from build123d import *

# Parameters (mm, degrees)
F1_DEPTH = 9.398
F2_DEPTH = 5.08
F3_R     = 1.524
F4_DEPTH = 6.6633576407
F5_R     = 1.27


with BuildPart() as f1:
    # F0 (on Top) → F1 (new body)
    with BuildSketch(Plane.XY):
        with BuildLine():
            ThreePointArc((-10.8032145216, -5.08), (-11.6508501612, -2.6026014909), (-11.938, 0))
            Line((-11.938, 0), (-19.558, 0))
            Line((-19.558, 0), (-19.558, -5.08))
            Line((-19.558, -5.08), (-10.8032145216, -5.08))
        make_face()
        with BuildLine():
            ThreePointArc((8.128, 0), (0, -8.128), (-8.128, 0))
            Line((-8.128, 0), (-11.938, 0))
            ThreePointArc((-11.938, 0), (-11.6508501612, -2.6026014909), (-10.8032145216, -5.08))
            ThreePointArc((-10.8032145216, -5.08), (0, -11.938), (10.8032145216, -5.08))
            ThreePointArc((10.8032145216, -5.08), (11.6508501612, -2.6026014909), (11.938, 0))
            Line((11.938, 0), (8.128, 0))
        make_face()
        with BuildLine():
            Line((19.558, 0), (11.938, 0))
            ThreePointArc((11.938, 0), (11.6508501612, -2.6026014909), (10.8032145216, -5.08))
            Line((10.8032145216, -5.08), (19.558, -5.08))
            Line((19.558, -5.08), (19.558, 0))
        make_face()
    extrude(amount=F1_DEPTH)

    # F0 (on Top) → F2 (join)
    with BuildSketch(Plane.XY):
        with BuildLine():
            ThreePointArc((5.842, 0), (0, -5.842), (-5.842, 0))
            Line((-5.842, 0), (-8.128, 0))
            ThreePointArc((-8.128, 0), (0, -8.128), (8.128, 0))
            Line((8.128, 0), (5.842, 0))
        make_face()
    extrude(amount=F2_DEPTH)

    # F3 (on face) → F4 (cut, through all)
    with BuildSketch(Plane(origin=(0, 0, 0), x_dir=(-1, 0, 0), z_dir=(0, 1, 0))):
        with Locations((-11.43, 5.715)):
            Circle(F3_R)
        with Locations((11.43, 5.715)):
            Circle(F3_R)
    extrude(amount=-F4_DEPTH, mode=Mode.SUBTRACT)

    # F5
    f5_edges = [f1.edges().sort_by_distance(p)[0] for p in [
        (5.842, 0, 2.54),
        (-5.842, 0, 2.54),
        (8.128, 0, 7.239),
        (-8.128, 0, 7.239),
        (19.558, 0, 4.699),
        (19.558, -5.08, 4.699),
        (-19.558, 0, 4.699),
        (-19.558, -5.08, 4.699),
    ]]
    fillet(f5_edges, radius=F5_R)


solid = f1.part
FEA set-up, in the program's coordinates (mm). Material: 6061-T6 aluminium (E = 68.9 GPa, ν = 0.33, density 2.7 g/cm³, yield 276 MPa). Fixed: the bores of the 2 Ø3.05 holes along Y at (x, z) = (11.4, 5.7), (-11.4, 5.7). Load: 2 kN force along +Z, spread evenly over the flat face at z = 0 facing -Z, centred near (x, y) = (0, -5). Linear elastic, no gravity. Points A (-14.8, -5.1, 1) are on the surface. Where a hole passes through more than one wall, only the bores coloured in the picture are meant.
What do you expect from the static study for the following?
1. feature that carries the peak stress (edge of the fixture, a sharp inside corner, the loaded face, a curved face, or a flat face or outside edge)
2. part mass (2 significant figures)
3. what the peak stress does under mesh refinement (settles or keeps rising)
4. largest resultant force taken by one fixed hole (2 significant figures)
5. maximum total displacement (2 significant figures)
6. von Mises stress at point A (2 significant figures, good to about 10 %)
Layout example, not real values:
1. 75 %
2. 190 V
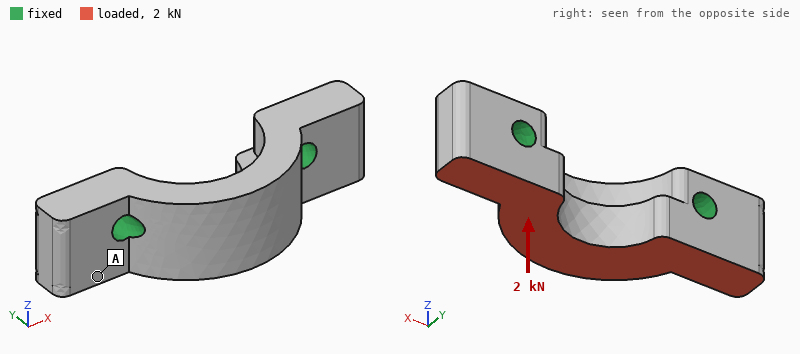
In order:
1. edge of the fixture
2. 5.5 g
3. keeps rising
4. 1.0 kN
5. 12 µm
6. 12 MPa
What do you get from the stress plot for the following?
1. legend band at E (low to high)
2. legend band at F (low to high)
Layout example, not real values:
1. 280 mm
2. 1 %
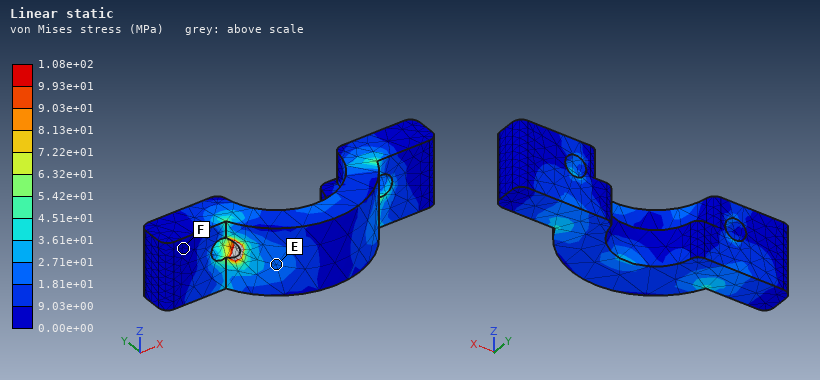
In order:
1. 1.81e+01 to 2.71e+01 MPa
2. 0.00e+00 to 9.03e+00 MPa
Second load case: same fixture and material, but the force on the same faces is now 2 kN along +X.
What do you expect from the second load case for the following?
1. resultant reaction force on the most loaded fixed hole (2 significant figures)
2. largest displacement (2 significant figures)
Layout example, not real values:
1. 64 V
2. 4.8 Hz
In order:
1. 1.1 kN
2. 9.3 µm
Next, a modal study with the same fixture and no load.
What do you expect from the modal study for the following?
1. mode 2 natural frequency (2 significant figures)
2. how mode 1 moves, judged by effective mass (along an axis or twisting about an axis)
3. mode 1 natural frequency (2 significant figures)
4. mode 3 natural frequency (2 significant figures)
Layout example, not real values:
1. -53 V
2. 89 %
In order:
1. 52 kHz
2. along Z
3. 31 kHz
4. 53 kHz
